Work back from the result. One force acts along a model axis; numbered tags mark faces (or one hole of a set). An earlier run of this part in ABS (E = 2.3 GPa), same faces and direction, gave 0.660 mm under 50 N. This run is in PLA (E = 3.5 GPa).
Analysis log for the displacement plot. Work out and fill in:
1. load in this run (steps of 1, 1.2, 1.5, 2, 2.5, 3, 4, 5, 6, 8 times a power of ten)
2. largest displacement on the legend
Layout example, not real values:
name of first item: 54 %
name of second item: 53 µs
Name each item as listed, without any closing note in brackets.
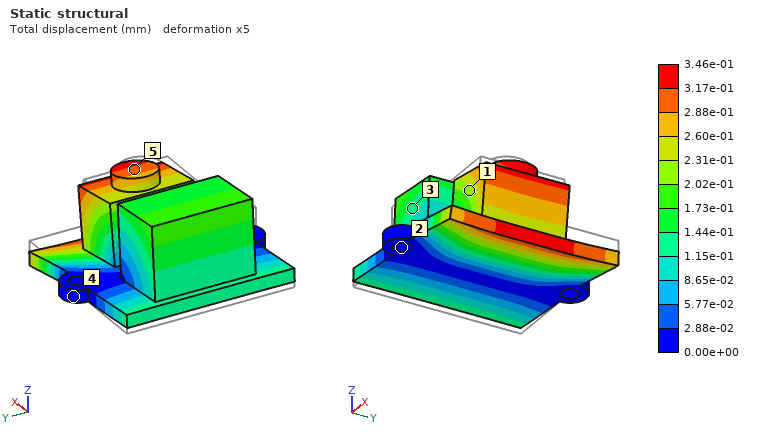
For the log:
load in this run: 40 N
largest displacement on the legend: 3.46e-01 mm
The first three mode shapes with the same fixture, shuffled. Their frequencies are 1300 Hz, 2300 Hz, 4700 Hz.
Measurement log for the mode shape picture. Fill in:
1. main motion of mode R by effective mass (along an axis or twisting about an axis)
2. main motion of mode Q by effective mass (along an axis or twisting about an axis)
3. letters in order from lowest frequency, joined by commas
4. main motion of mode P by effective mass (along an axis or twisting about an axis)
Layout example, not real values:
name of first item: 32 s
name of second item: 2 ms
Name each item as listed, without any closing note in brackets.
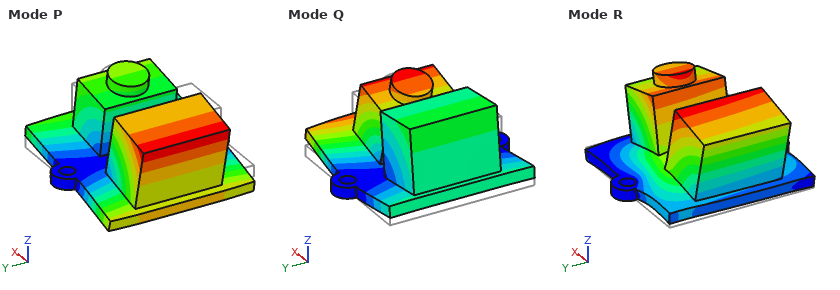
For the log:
main motion of mode R by effective mass: along Z
main motion of mode Q by effective mass: along Z
letters in order from lowest frequency, joined by commas: P, Q, R
main motion of mode P by effective mass: along X
